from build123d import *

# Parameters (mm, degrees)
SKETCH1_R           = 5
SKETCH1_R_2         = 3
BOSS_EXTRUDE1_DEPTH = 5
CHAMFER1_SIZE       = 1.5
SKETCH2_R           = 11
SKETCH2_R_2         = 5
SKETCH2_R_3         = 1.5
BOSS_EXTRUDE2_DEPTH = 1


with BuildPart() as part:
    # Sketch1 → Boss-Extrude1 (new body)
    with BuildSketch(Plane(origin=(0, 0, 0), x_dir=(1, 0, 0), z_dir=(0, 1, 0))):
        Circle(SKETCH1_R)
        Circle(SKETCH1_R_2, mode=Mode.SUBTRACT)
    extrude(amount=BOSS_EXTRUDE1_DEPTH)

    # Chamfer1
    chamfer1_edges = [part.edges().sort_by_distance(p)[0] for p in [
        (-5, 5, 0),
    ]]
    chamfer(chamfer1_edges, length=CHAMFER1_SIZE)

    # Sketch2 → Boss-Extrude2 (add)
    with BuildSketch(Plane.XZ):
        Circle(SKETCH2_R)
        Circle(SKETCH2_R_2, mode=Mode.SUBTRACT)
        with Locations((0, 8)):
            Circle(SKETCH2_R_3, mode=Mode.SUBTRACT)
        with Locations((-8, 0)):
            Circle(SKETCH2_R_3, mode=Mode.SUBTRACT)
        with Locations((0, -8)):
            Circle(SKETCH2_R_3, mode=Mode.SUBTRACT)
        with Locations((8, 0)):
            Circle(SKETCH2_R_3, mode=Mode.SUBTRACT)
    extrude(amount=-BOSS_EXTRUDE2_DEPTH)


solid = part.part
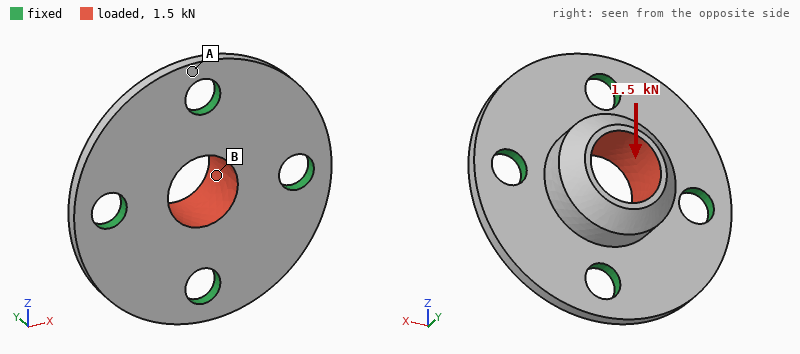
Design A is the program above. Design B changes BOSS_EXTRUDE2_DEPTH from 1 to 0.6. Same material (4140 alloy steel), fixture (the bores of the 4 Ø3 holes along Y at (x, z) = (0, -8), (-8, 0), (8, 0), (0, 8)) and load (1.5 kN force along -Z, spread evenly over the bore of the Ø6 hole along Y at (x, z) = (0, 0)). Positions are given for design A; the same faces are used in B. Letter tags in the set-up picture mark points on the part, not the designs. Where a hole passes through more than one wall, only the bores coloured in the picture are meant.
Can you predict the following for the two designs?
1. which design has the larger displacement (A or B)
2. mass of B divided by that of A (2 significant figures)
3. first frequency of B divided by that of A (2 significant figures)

B
0.78
0.63
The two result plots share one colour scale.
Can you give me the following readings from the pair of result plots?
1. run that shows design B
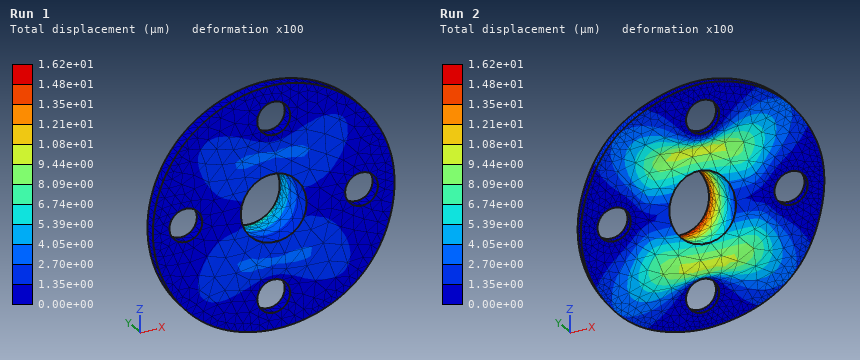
Run 2
